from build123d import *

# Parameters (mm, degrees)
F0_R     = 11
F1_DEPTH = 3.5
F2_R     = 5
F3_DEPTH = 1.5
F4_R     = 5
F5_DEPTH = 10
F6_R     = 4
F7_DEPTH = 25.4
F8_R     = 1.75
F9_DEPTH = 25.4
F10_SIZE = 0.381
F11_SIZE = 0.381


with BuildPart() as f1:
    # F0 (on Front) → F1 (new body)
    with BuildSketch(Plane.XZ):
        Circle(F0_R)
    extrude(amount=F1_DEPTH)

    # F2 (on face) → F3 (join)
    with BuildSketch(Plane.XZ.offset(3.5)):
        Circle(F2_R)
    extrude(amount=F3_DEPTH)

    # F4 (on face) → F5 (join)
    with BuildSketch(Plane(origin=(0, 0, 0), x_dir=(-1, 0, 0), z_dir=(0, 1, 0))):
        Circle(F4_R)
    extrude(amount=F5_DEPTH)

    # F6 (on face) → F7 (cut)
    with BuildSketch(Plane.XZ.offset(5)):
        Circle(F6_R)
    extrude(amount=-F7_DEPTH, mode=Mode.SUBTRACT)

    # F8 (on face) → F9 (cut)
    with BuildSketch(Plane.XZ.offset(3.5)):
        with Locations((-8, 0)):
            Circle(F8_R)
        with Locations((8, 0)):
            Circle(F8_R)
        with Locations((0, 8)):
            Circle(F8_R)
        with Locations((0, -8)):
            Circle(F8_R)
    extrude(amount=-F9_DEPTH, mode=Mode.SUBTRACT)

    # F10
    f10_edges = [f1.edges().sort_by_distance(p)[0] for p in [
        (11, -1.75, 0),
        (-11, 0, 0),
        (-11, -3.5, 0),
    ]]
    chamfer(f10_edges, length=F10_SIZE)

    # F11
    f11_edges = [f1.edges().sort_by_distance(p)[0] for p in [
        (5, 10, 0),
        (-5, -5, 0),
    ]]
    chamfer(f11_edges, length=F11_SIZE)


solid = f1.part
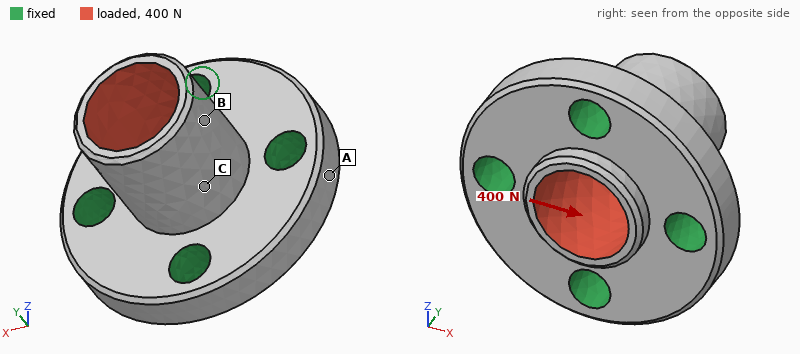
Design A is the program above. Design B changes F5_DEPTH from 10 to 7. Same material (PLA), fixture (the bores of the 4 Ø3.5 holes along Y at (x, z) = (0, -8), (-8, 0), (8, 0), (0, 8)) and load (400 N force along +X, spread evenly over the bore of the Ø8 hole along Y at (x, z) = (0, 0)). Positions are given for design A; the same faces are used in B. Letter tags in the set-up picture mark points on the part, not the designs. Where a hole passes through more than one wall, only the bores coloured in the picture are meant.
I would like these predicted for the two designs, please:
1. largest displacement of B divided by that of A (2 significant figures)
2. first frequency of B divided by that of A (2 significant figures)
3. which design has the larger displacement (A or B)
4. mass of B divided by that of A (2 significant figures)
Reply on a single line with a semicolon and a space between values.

0.56; 1.3; A; 0.94
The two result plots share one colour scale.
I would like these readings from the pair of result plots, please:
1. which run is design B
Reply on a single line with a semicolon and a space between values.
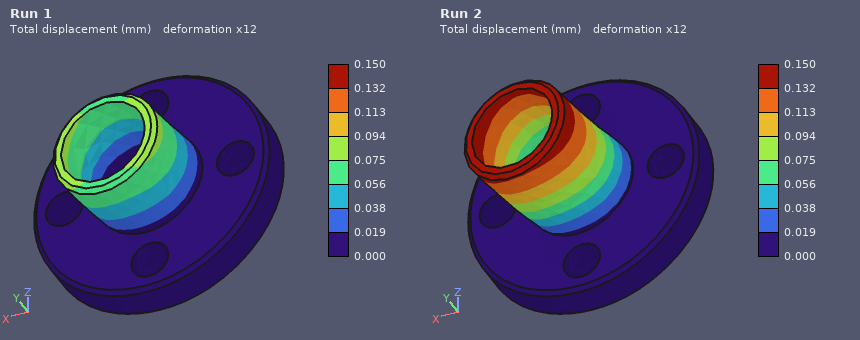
Run 1
